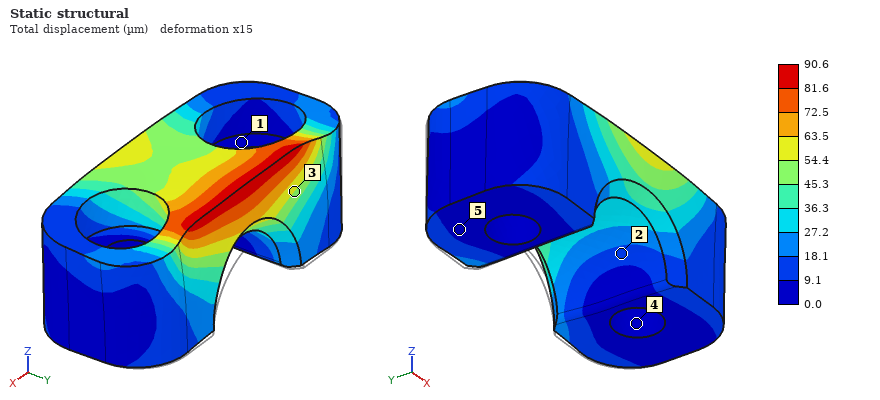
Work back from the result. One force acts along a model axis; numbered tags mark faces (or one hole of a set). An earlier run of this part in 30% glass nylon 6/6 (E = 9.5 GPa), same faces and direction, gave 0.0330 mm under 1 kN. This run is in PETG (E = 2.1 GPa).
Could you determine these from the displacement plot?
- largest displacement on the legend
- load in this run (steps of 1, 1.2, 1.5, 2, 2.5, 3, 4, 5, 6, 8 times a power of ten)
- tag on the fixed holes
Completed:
90.6 µm
600 N
4
